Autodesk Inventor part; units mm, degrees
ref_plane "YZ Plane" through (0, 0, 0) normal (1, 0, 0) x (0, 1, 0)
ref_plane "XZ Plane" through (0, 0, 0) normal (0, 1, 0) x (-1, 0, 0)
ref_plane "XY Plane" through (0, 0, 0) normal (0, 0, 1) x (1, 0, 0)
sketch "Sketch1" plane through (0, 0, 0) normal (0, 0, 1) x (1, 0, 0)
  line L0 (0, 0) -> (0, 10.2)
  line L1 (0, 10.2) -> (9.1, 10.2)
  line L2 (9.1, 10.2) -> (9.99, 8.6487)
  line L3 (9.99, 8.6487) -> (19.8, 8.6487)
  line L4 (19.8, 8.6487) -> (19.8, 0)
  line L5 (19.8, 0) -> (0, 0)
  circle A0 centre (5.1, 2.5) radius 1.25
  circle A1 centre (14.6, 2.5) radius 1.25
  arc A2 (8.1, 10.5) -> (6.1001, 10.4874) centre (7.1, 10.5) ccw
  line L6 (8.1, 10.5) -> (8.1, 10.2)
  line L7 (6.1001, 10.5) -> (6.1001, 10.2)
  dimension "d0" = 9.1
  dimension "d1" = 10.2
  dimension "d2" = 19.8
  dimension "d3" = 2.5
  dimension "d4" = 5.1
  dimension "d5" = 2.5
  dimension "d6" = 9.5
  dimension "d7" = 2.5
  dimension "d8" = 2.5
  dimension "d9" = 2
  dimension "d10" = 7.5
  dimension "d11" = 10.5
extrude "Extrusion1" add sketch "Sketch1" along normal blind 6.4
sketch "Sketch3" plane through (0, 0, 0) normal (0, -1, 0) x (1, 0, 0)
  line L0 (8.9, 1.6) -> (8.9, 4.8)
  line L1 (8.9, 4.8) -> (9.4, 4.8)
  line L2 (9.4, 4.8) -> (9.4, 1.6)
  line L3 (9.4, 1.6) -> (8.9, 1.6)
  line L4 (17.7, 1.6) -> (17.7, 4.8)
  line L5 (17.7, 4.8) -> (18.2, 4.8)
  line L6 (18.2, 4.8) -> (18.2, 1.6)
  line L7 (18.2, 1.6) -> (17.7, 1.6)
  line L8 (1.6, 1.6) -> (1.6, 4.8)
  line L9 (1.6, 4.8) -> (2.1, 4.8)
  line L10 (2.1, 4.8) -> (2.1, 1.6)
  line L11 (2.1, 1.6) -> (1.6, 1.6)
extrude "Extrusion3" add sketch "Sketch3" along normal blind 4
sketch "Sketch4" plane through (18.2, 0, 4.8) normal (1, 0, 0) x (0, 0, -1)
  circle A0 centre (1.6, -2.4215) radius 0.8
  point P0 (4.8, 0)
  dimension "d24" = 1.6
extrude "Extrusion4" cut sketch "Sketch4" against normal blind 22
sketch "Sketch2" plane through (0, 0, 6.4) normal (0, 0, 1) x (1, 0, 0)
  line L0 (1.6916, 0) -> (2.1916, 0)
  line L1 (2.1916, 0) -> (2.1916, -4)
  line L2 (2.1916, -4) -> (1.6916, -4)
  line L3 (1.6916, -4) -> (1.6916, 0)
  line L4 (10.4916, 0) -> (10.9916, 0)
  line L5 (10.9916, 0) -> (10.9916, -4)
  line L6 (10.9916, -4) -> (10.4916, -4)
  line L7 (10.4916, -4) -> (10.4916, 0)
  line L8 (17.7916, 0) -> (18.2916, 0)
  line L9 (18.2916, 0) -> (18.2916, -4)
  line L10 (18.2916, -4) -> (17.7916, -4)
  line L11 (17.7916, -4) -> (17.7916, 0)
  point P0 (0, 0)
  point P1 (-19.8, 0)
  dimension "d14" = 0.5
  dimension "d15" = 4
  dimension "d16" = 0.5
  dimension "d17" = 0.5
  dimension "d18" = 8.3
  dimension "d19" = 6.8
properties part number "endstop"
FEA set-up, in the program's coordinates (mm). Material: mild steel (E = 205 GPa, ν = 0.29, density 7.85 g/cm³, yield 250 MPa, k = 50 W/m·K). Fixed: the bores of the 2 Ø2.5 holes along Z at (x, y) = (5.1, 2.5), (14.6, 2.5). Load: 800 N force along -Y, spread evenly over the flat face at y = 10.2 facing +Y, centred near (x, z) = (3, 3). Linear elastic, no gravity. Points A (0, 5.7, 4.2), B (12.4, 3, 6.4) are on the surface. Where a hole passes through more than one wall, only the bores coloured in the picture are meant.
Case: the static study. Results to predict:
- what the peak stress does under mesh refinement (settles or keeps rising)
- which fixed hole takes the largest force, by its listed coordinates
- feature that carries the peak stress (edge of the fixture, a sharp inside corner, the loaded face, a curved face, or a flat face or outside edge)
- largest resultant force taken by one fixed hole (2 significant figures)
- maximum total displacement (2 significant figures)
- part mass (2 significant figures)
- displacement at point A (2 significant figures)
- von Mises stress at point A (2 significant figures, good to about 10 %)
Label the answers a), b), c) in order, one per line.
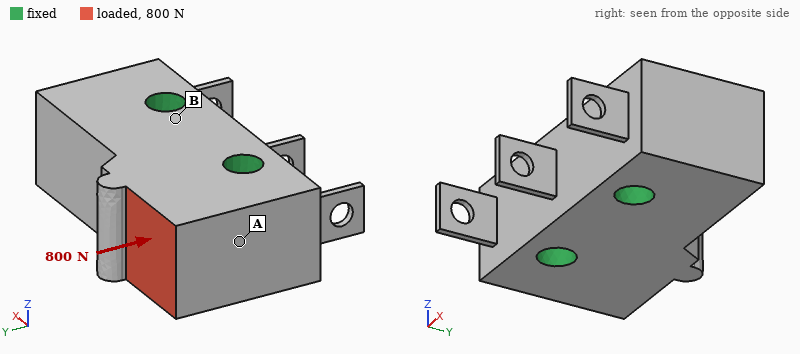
a) keeps rising
b) (5.1, 2.5)
c) edge of the fixture
d) 880 N
e) 1.6 µm
f) 9.1 g
g) 1.00 µm
h) 15 MPa
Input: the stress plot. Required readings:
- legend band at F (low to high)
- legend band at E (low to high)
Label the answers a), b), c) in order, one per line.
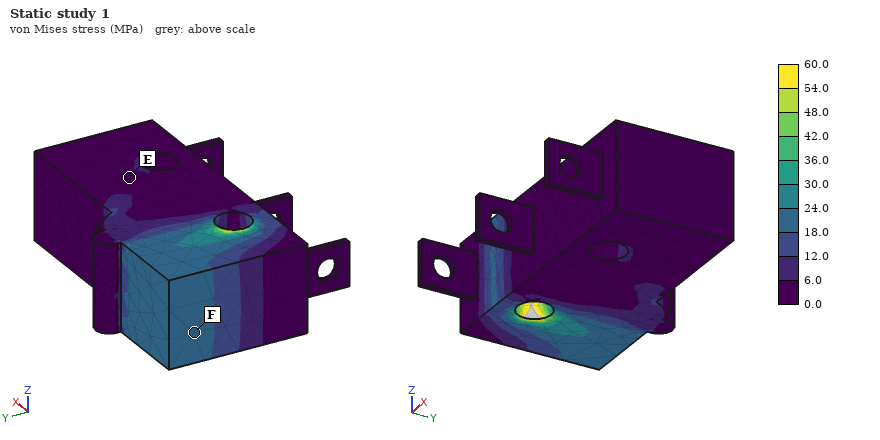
a) 18.0 to 24.0 MPa
b) 0.0 to 6.0 MPa
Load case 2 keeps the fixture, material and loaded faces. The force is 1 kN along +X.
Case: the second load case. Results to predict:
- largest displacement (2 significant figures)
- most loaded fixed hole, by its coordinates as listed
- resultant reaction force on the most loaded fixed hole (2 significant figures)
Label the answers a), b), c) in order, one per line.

a) 4.4 µm
b) (14.6, 2.5)
c) 830 N
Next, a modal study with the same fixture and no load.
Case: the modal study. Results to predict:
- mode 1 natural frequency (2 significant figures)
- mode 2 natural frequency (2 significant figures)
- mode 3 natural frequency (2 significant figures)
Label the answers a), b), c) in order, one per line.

a) 25 kHz
b) 25 kHz
c) 25 kHz
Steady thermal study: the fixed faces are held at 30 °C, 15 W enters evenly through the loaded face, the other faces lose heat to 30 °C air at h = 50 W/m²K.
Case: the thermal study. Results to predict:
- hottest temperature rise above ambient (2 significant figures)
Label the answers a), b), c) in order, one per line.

a) 46 K
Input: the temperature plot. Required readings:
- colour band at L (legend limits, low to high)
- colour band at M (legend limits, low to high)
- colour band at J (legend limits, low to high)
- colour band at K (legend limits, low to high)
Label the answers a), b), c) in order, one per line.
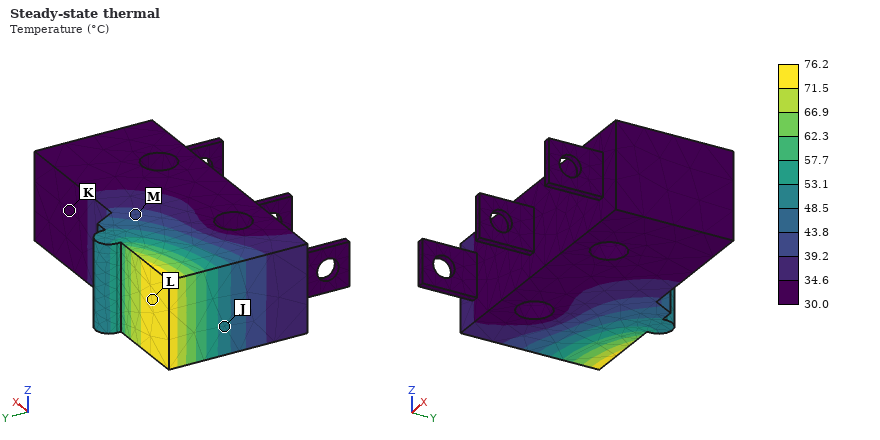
a) 71.5 to 76.2 °C
b) 39.2 to 43.8 °C
c) 48.5 to 53.1 °C
d) 30.0 to 34.6 °C
